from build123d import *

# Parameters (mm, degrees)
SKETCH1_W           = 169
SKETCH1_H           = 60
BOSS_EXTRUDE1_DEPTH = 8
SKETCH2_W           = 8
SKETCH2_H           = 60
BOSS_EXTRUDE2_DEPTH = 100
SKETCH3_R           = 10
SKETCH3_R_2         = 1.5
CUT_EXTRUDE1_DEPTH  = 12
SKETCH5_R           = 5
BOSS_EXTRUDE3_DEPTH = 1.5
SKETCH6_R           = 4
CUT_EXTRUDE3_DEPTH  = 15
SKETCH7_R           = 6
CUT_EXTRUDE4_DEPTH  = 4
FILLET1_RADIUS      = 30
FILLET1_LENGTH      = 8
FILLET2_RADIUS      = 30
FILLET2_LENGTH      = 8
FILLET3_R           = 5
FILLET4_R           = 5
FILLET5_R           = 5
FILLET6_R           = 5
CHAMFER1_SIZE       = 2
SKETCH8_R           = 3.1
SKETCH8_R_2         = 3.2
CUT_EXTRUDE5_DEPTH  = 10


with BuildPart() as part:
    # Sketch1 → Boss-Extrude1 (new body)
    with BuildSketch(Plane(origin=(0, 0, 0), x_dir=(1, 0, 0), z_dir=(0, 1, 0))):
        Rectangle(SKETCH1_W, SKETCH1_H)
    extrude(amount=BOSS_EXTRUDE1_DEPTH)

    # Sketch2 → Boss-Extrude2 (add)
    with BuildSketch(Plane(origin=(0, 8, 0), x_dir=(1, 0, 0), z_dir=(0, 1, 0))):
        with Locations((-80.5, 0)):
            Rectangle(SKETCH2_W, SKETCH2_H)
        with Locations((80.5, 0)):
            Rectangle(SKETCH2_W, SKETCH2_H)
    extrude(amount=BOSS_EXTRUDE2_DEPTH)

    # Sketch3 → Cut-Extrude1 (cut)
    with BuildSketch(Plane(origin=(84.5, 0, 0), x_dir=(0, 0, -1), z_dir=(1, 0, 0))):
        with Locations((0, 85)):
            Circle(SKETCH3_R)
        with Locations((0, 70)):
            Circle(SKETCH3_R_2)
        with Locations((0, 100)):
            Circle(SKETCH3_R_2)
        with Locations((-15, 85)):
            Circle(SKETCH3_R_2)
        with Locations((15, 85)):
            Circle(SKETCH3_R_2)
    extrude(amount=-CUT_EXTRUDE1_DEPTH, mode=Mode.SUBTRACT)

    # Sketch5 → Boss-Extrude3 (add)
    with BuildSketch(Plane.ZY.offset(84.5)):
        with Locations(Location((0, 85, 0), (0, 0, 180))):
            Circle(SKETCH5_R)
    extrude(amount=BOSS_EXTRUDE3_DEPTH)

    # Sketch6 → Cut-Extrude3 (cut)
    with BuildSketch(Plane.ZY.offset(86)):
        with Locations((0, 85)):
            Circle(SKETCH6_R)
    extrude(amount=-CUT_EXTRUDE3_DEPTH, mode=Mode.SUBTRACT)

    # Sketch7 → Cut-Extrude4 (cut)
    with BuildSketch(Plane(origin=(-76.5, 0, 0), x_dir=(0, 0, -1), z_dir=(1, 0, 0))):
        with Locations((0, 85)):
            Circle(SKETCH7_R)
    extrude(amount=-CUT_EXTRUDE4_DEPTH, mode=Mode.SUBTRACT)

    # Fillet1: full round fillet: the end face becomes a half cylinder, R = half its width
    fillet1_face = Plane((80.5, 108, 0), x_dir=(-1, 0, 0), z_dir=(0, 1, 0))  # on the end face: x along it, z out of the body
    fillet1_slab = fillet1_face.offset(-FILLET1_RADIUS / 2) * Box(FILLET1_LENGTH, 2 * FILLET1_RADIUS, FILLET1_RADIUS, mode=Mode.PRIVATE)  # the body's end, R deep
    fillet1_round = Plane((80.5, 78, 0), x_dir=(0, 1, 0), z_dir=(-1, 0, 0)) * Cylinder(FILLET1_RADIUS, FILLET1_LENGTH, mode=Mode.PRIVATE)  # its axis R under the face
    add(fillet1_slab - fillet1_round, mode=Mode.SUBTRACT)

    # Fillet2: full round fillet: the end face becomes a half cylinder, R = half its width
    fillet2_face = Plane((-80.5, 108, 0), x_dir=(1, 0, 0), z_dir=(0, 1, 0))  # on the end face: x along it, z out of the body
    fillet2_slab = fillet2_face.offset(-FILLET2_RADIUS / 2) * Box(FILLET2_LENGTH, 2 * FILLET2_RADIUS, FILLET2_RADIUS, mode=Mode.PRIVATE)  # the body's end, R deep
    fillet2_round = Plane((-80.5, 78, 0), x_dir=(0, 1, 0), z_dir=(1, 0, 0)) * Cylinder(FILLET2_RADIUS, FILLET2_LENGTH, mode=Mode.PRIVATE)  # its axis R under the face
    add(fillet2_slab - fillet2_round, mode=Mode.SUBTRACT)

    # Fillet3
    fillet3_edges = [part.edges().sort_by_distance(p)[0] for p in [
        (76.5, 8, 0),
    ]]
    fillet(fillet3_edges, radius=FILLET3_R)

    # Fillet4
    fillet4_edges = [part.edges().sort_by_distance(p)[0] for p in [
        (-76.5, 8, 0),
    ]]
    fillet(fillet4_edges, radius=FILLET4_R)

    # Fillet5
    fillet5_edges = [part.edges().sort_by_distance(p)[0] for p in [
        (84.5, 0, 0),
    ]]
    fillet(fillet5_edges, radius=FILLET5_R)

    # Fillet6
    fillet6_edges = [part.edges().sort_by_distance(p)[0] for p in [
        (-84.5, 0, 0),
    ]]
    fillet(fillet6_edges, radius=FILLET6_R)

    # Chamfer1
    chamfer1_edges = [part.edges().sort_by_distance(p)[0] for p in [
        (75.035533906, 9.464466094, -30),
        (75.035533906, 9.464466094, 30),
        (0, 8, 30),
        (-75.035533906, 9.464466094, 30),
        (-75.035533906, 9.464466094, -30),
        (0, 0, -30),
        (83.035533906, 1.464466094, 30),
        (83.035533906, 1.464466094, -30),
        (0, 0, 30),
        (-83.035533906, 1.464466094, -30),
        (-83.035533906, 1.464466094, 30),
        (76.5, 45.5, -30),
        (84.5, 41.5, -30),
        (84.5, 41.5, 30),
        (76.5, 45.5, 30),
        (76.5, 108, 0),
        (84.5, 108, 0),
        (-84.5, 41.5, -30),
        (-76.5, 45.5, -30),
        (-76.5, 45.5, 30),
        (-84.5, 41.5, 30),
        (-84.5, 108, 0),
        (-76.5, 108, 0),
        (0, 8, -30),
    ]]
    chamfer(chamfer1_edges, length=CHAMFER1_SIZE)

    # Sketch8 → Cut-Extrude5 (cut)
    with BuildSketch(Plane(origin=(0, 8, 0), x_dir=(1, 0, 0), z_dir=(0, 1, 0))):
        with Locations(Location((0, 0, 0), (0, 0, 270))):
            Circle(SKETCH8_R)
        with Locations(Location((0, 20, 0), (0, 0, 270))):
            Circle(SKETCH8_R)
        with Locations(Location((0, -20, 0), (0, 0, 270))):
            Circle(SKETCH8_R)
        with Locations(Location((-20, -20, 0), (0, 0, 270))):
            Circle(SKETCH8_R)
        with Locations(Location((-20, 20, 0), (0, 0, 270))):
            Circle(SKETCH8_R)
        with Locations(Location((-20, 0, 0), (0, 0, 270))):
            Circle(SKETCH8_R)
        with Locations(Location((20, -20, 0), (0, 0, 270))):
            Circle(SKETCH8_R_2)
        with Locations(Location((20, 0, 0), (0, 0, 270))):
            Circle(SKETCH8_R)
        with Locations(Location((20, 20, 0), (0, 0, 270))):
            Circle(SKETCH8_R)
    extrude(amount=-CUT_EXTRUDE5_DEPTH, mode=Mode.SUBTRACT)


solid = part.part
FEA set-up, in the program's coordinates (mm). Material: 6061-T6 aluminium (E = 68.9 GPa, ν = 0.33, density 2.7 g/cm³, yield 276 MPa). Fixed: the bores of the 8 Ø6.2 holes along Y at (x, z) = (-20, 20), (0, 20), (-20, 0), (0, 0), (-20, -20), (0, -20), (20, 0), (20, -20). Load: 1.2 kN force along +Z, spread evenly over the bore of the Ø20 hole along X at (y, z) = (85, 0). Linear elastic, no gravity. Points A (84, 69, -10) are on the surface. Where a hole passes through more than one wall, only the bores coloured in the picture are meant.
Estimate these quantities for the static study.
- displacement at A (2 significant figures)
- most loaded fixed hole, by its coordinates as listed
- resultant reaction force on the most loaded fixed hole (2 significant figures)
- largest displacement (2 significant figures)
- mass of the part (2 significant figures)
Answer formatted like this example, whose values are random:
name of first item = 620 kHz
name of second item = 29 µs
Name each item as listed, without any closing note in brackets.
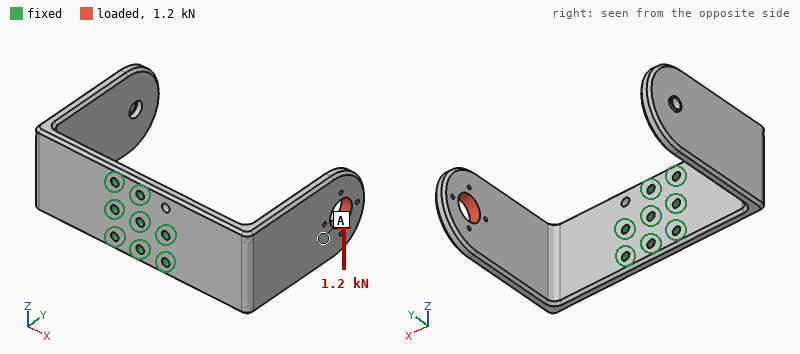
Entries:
displacement at A = 1.1 mm
most loaded fixed hole, by its coordinates as listed = (20, -20)
resultant reaction force on the most loaded fixed hole = 3.4 kN
largest displacement = 1.9 mm
mass of the part = 440 g
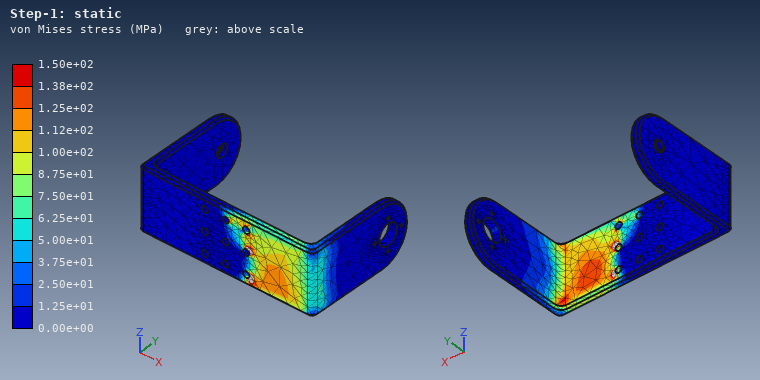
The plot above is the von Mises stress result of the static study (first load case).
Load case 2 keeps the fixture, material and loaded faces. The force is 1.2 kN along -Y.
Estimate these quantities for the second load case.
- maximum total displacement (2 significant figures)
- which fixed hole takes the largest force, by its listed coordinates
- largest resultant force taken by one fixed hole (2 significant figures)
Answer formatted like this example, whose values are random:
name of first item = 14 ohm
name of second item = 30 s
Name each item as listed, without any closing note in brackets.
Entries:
maximum total displacement = 1.4 mm
which fixed hole takes the largest force, by its listed coordinates = (20, 0)
largest resultant force taken by one fixed hole = 2.1 kN
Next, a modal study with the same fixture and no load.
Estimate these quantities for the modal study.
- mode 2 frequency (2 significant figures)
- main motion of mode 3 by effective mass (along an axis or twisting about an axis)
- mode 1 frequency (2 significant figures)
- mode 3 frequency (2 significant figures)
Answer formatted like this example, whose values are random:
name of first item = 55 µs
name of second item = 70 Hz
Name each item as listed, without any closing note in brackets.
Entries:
mode 2 frequency = 370 Hz
main motion of mode 3 by effective mass = along Z
mode 1 frequency = 360 Hz
mode 3 frequency = 590 Hz
